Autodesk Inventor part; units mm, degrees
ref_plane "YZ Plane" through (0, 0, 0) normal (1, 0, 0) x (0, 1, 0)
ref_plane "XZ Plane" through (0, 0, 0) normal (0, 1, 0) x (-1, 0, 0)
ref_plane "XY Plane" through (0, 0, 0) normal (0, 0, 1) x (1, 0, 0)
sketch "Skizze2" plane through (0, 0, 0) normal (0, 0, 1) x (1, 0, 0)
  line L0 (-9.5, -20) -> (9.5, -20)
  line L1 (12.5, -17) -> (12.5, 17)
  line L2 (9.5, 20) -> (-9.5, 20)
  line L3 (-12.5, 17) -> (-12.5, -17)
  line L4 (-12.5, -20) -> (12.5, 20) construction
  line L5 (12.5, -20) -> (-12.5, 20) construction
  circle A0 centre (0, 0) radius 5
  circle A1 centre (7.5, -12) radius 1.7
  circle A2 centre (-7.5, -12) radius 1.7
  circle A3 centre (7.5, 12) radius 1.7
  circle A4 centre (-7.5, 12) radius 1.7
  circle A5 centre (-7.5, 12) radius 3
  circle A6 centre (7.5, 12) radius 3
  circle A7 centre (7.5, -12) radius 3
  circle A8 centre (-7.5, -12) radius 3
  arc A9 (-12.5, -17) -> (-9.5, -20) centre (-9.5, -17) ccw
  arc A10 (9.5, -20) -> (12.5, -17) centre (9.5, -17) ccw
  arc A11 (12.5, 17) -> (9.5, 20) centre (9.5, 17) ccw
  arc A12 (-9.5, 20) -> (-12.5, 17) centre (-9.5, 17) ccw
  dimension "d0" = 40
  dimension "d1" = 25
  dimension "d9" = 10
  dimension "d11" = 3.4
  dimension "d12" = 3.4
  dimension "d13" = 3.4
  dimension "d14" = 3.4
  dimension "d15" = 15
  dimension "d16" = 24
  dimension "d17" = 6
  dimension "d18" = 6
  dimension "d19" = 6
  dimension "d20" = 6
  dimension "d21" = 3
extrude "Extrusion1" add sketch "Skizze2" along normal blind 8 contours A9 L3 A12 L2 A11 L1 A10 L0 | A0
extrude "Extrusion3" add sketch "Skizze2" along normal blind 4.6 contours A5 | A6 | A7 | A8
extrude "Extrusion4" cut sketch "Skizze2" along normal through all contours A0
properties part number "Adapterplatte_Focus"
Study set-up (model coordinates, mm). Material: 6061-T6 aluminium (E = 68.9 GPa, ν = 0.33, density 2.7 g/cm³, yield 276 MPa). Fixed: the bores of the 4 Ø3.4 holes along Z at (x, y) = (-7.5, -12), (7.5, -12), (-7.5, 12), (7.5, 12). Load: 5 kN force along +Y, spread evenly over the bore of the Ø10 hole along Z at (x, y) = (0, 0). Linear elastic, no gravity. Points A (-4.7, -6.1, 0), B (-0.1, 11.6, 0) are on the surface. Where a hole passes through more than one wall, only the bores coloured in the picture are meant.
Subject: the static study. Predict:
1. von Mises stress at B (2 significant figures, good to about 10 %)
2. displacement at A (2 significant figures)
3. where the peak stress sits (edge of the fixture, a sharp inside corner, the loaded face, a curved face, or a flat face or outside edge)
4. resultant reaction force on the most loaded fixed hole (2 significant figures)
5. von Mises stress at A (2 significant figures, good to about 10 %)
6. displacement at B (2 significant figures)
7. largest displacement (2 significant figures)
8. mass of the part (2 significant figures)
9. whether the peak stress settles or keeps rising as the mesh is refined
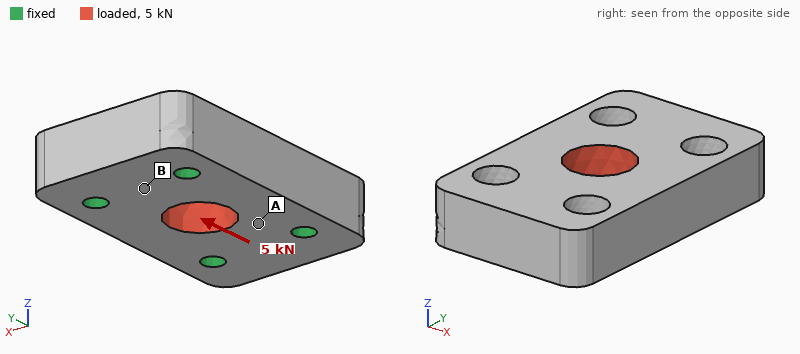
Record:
9.9 MPa
2.0 µm
edge of the fixture
1.3 kN
24 MPa
1.7 µm
4.5 µm
18 g
keeps rising
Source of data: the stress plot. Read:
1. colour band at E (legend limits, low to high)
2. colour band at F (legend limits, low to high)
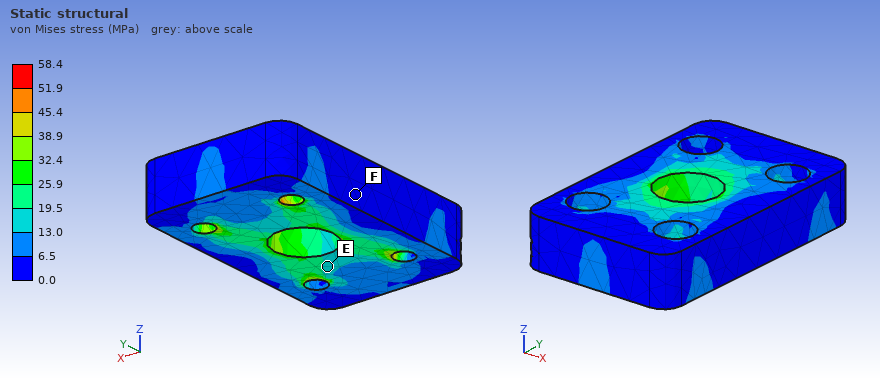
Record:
13.0 to 19.5 MPa
0.0 to 6.5 MPa
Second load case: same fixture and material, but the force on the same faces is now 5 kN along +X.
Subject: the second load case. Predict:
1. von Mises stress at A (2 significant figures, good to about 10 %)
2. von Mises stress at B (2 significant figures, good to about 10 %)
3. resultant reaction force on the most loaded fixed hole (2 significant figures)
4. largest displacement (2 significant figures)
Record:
23 MPa
16 MPa
1.4 kN
8.3 µm
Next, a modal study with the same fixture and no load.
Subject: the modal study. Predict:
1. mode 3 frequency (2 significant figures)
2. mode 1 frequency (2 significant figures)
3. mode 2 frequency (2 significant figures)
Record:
43 kHz
36 kHz
43 kHz
